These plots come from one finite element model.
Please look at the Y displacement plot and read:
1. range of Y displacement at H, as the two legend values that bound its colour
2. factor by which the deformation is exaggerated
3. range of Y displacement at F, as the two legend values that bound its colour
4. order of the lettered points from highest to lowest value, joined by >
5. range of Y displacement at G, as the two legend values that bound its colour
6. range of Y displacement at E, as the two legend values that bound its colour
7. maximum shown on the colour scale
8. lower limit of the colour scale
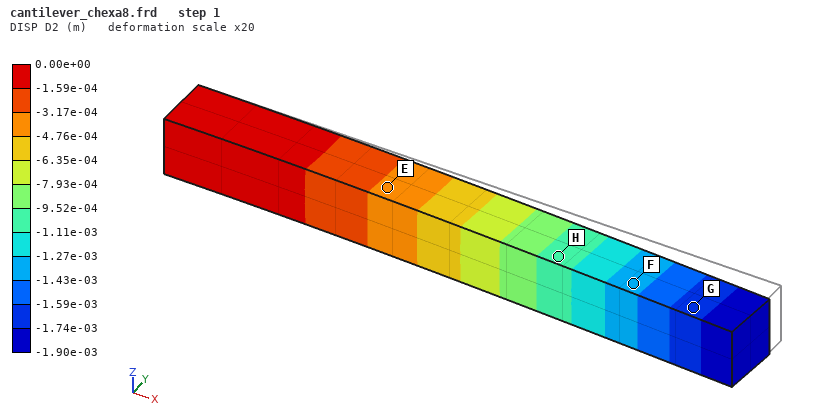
-1.11e-03 to -9.52e-04 m
20
-1.43e-03 to -1.27e-03 m
E > H > F > G
-1.74e-03 to -1.59e-03 m
-4.76e-04 to -3.17e-04 m
0.00e+00 m
-1.90e-03 m
